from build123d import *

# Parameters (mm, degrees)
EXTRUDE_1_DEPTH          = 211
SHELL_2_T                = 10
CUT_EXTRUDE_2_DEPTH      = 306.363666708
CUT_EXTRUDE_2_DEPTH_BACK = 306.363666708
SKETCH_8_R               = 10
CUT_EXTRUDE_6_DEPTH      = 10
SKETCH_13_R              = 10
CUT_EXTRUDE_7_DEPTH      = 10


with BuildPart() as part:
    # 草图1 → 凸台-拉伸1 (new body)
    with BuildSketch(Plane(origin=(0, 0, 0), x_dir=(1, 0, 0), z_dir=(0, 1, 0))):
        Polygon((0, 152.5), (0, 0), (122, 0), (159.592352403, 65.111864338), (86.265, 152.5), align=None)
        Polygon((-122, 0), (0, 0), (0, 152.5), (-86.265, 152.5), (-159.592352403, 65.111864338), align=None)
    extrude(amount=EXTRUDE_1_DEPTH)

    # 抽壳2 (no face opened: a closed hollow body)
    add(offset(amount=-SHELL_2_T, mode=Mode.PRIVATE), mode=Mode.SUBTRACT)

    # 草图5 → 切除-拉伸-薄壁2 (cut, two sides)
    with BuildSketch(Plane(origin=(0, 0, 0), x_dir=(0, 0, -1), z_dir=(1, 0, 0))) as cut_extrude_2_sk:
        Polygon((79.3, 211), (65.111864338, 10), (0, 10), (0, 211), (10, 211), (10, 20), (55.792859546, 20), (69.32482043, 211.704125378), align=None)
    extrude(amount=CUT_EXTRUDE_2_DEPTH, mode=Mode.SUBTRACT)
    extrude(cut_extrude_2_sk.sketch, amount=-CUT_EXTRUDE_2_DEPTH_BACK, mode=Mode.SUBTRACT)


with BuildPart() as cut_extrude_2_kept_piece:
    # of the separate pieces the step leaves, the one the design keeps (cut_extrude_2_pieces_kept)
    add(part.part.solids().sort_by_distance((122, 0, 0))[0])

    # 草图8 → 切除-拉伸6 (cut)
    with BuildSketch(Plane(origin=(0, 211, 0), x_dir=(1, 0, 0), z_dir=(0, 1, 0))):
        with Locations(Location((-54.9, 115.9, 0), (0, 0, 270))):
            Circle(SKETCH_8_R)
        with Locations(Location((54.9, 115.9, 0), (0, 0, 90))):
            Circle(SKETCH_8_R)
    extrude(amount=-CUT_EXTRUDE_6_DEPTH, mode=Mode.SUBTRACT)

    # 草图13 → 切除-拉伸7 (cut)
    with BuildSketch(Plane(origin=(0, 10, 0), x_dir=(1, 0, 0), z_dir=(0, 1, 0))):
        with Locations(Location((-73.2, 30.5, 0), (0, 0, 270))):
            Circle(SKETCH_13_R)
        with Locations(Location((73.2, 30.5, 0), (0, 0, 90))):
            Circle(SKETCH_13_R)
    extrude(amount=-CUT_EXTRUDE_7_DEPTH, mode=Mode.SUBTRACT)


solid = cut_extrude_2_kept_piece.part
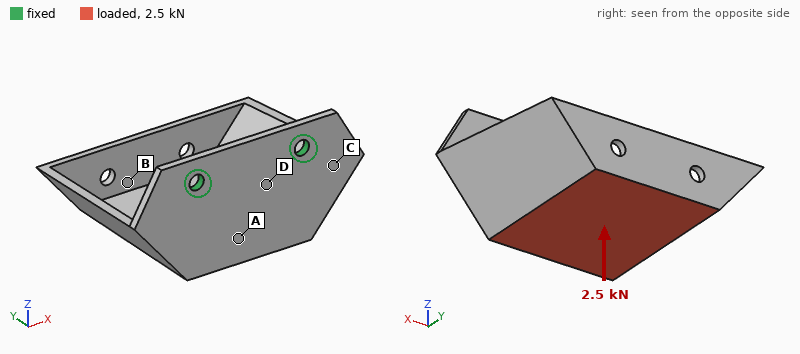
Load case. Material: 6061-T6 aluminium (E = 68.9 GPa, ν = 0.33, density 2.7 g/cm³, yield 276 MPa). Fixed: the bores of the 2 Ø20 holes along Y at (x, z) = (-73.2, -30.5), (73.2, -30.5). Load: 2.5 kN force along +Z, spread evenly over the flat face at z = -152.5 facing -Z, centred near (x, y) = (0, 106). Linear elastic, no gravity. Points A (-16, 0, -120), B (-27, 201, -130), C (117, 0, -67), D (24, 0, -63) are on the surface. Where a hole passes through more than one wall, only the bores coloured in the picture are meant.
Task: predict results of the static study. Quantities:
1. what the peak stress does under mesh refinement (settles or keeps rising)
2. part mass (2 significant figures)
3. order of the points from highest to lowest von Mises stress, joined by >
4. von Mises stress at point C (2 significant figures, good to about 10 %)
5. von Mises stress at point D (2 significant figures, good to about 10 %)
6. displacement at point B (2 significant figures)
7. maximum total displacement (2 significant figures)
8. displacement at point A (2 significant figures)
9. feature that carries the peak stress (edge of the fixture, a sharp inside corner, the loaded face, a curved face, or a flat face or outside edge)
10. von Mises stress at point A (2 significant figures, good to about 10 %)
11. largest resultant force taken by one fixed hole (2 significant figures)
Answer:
keeps rising
3.4 kg
C > D > A > B
53 MPa
35 MPa
2.4 mm
2.6 mm
0.58 mm
edge of the fixture
21 MPa
1.3 kN
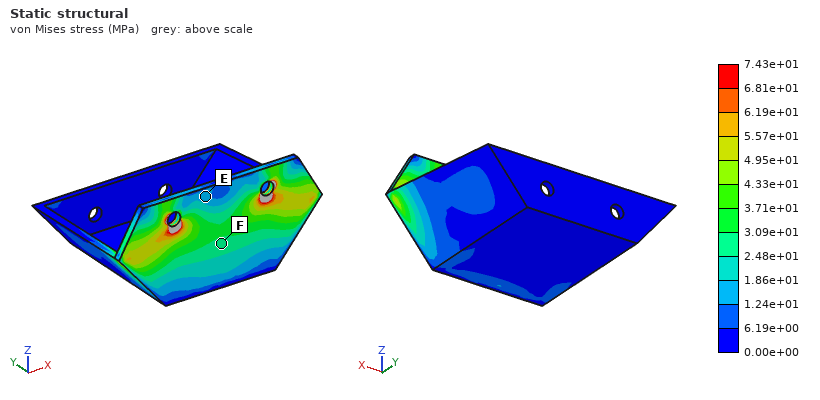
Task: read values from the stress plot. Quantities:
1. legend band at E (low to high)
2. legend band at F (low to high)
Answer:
1.24e+01 to 1.86e+01 MPa
2.48e+01 to 3.09e+01 MPa
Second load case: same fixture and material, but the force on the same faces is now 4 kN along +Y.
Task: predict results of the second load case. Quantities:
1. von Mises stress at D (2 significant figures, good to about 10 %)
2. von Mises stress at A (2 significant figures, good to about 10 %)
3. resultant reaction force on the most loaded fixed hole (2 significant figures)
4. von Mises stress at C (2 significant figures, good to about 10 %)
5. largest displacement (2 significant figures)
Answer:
54 MPa
16 MPa
2.0 kN
64 MPa
3.4 mm
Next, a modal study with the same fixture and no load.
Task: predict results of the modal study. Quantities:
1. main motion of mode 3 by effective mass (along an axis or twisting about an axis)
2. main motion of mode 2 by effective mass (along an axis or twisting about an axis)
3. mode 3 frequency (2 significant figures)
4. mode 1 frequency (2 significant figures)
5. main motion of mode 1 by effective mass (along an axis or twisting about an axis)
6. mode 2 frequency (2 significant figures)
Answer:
along Y
along X
440 Hz
100 Hz
along Z
180 Hz
